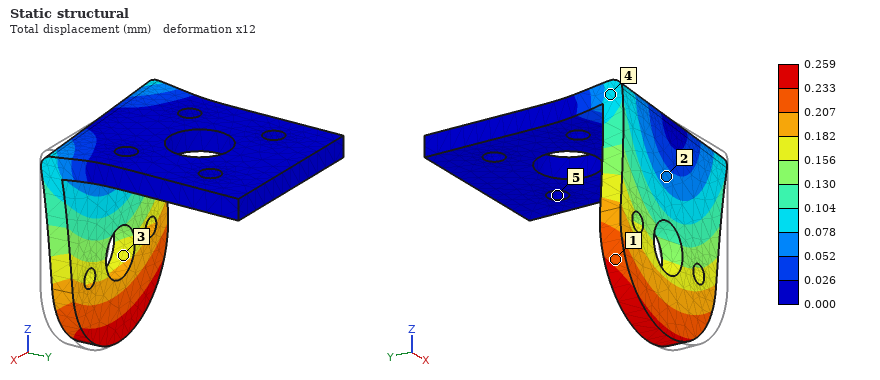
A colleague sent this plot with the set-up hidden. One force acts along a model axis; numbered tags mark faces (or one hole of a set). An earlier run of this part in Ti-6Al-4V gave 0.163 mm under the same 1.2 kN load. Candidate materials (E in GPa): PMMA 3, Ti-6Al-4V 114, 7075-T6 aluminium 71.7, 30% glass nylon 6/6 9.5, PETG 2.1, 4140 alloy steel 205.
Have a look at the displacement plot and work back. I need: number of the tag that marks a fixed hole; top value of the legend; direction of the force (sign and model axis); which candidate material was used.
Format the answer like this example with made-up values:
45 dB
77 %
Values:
5
0.259 mm
-X
7075-T6 aluminium
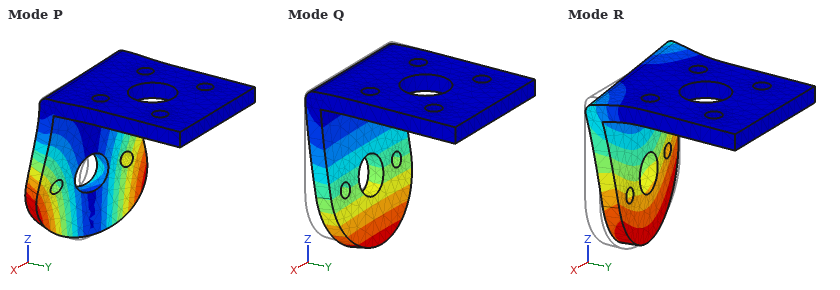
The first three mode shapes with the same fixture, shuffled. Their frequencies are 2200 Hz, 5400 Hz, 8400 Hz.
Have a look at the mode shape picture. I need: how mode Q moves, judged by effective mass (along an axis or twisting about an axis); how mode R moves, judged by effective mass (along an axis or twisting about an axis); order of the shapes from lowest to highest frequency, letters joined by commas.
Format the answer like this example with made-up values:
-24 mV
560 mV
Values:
along Y
along X
Q, R, P
